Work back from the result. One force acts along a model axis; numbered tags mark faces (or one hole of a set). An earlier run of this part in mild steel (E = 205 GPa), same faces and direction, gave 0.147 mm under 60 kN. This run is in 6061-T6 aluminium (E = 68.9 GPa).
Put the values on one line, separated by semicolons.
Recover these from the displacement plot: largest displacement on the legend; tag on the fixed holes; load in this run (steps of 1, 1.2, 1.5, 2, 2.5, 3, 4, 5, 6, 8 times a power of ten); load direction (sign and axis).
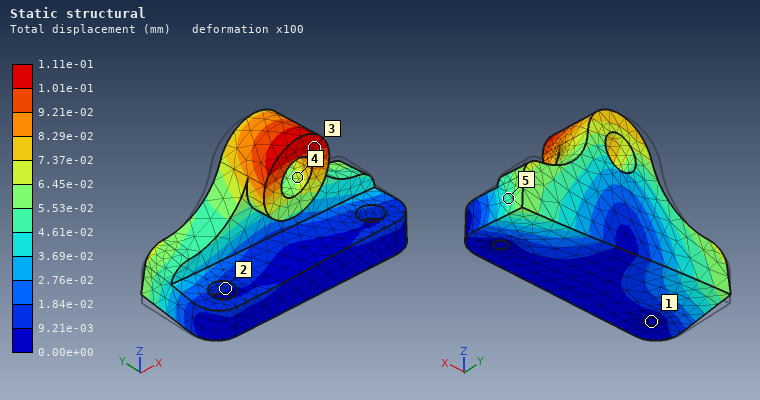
1.11e-01 mm; 1; 15 kN; +X
